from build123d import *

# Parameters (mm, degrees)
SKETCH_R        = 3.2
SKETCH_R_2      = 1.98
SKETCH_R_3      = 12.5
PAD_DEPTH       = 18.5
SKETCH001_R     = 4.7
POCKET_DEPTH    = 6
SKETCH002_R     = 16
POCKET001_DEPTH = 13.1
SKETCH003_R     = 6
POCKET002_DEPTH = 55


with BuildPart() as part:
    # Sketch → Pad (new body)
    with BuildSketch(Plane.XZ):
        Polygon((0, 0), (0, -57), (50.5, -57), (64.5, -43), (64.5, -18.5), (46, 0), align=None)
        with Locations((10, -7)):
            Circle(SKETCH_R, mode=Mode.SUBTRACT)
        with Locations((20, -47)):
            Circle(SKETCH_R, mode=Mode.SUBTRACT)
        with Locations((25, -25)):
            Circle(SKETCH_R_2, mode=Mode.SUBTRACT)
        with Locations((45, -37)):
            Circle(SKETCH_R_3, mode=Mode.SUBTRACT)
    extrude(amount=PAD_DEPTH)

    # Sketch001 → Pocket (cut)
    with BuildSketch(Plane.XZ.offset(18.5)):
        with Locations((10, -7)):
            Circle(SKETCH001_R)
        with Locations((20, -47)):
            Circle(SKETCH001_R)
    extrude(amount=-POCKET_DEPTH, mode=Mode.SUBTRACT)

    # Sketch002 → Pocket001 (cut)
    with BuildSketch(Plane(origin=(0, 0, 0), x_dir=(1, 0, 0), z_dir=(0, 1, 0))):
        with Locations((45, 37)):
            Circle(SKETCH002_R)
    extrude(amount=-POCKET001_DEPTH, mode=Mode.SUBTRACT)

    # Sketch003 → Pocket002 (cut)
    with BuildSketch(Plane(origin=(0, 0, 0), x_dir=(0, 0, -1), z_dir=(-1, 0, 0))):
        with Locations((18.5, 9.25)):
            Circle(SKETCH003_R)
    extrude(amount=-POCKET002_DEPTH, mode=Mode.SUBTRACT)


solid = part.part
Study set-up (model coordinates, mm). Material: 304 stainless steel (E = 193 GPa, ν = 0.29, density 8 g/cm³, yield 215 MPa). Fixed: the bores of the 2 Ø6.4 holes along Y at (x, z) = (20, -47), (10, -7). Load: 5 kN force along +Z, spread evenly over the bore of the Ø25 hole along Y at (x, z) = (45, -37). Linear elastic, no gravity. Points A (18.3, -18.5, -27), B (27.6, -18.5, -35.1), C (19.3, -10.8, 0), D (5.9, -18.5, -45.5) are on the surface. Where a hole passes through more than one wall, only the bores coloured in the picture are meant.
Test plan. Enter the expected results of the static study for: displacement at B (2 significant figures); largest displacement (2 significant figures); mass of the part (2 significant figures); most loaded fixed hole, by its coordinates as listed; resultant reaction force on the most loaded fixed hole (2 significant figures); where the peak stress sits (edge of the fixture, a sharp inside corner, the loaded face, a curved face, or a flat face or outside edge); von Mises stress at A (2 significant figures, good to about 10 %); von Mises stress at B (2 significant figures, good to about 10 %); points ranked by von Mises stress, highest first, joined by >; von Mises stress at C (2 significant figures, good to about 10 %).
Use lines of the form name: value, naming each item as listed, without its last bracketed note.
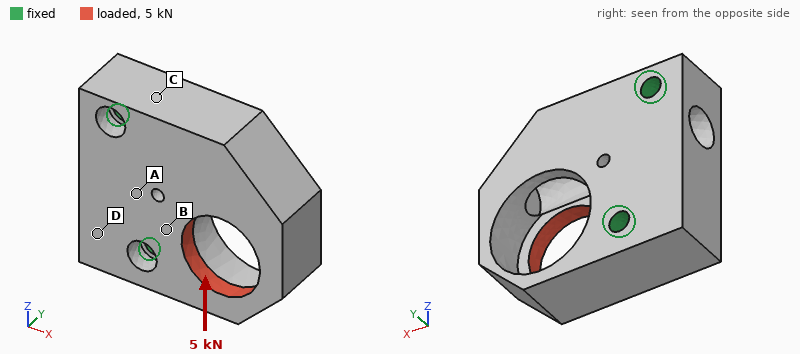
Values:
displacement at B: 3.1 µm
largest displacement: 20 µm
mass of the part: 340 g
most loaded fixed hole, by its coordinates as listed: (20, -47)
resultant reaction force on the most loaded fixed hole: 5.1 kN
where the peak stress sits: edge of the fixture
von Mises stress at A: 12 MPa
von Mises stress at B: 34 MPa
points ranked by von Mises stress, highest first, joined by >: B > C > A > D
von Mises stress at C: 22 MPa
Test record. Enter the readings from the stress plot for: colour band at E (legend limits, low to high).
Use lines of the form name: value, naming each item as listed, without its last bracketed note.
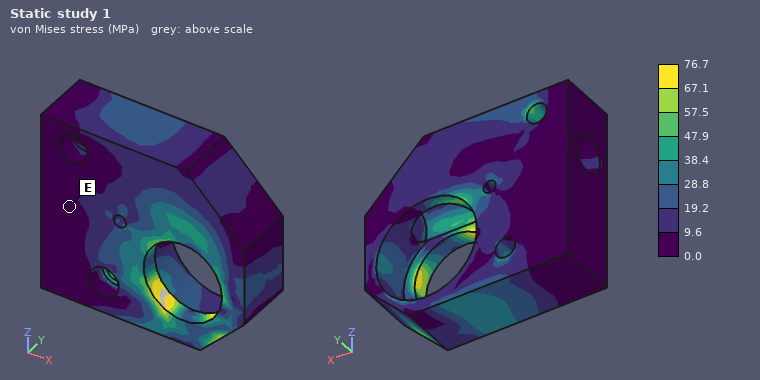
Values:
colour band at E: 0.0 to 9.6 MPa
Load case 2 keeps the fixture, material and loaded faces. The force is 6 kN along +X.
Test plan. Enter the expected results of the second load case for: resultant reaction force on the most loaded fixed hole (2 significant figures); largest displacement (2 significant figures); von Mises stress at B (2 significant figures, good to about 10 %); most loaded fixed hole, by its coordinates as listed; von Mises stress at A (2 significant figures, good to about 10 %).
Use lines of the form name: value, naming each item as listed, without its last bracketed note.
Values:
resultant reaction force on the most loaded fixed hole: 4.3 kN
largest displacement: 23 µm
von Mises stress at B: 20 MPa
most loaded fixed hole, by its coordinates as listed: (20, -47)
von Mises stress at A: 10 MPa
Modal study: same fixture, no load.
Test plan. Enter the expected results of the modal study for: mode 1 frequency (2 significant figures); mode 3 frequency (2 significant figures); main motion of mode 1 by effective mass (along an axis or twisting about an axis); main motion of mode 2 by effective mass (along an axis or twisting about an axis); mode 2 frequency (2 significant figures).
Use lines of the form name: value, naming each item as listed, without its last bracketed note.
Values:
mode 1 frequency: 4700 Hz
mode 3 frequency: 11 kHz
main motion of mode 1 by effective mass: along Y
main motion of mode 2 by effective mass: along Z
mode 2 frequency: 8400 Hz
